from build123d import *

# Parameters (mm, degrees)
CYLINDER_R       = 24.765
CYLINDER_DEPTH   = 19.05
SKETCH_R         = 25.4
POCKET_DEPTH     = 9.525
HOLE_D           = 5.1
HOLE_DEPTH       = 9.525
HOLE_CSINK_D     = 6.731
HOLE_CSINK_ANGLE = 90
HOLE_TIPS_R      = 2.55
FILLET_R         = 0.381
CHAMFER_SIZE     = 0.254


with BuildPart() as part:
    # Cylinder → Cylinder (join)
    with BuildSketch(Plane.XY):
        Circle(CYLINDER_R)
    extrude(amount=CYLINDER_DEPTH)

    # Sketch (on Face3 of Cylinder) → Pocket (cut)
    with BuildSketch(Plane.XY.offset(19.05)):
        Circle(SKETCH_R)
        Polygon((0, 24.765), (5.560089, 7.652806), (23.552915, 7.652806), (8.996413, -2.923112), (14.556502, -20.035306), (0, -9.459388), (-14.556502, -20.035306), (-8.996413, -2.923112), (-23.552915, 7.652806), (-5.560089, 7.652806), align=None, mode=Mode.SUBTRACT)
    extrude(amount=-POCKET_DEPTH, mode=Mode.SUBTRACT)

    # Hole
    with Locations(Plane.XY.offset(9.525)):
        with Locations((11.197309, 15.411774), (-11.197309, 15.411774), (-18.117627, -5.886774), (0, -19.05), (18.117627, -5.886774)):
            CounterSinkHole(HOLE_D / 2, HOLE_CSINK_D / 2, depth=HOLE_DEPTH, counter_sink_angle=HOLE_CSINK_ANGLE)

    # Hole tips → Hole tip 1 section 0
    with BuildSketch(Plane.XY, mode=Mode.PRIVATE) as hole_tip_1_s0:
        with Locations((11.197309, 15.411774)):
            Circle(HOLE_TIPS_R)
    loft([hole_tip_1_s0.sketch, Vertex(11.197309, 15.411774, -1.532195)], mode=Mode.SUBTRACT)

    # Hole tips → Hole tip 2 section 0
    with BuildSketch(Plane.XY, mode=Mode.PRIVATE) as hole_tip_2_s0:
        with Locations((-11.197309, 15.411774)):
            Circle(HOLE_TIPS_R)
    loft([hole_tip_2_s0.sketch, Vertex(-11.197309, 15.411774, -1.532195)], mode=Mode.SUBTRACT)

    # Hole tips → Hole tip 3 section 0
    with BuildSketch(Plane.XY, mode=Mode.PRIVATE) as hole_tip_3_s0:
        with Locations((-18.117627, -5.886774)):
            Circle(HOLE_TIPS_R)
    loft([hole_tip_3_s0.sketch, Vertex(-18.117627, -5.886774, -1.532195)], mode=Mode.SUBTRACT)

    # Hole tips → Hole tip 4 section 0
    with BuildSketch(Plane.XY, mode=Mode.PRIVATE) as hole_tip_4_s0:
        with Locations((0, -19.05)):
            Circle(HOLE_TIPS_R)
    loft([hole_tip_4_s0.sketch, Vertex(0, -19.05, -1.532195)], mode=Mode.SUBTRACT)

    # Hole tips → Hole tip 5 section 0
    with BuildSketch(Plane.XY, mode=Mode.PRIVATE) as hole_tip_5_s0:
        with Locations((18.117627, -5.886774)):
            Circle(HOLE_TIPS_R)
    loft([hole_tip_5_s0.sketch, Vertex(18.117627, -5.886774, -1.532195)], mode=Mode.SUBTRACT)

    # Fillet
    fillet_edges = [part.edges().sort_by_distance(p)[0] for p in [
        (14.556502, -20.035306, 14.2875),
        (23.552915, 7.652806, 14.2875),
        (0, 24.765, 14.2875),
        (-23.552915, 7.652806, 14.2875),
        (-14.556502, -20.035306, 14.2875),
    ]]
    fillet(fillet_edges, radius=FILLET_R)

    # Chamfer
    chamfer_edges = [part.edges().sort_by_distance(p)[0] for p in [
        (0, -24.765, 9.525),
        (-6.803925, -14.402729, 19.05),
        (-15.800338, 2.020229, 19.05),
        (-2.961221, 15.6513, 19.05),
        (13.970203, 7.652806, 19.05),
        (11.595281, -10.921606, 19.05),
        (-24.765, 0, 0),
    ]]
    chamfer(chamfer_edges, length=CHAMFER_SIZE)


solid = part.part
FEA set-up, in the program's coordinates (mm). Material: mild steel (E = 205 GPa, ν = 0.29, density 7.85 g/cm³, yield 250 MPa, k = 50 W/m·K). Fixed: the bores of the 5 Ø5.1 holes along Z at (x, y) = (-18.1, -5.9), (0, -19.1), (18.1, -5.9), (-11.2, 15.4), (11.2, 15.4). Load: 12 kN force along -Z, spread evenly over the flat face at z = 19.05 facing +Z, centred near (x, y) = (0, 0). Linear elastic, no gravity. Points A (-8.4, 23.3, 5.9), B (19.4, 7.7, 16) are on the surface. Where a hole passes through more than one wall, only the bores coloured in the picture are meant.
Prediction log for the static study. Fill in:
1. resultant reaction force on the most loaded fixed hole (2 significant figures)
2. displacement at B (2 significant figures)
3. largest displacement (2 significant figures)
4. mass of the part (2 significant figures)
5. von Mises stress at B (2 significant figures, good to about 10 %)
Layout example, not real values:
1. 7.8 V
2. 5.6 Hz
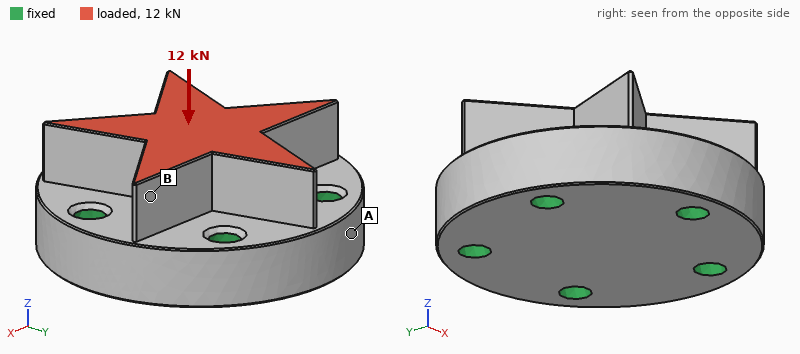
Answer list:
1. 2.5 kN
2. 1.9 µm
3. 3.1 µm
4. 190 g
5. 16 MPa
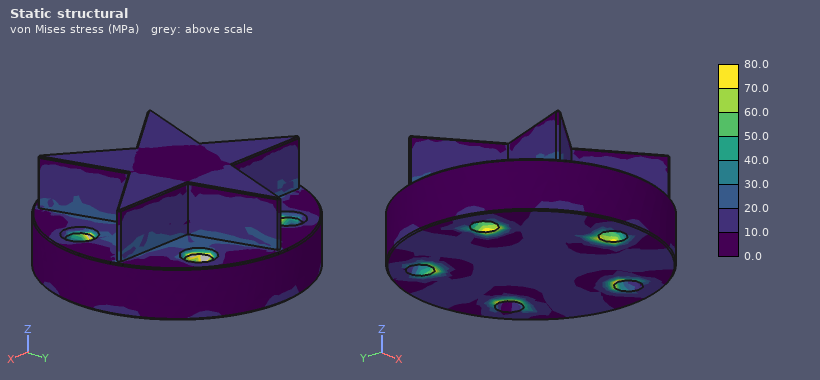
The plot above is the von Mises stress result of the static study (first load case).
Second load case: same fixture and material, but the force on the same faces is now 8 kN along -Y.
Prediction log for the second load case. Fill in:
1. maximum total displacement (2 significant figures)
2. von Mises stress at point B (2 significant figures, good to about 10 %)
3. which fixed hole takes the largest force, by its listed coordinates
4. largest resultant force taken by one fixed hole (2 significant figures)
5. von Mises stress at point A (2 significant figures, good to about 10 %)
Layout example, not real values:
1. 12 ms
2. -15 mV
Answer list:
1. 7.6 µm
2. 25 MPa
3. (0, -19.1)
4. 3.2 kN
5. 16 MPa
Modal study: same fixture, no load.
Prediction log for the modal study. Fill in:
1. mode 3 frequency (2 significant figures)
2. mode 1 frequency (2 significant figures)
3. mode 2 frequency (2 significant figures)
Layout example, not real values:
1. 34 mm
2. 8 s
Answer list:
1. 36 kHz
2. 35 kHz
3. 36 kHz
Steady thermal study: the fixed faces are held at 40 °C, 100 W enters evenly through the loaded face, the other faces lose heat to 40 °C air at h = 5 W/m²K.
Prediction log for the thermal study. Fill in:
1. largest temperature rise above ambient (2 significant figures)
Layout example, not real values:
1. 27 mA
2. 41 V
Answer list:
1. 54 K
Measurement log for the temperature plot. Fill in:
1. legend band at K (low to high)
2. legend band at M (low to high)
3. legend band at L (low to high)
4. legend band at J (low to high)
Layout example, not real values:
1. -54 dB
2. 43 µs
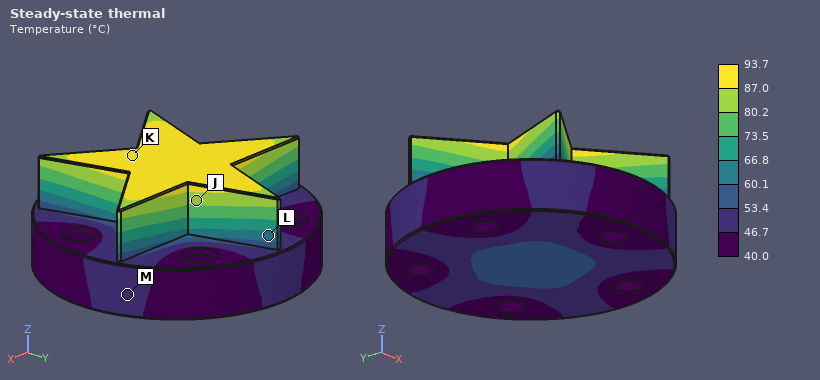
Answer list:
1. 87.0 to 93.7 °C
2. 46.7 to 53.4 °C
3. 60.1 to 66.8 °C
4. 80.2 to 87.0 °C
